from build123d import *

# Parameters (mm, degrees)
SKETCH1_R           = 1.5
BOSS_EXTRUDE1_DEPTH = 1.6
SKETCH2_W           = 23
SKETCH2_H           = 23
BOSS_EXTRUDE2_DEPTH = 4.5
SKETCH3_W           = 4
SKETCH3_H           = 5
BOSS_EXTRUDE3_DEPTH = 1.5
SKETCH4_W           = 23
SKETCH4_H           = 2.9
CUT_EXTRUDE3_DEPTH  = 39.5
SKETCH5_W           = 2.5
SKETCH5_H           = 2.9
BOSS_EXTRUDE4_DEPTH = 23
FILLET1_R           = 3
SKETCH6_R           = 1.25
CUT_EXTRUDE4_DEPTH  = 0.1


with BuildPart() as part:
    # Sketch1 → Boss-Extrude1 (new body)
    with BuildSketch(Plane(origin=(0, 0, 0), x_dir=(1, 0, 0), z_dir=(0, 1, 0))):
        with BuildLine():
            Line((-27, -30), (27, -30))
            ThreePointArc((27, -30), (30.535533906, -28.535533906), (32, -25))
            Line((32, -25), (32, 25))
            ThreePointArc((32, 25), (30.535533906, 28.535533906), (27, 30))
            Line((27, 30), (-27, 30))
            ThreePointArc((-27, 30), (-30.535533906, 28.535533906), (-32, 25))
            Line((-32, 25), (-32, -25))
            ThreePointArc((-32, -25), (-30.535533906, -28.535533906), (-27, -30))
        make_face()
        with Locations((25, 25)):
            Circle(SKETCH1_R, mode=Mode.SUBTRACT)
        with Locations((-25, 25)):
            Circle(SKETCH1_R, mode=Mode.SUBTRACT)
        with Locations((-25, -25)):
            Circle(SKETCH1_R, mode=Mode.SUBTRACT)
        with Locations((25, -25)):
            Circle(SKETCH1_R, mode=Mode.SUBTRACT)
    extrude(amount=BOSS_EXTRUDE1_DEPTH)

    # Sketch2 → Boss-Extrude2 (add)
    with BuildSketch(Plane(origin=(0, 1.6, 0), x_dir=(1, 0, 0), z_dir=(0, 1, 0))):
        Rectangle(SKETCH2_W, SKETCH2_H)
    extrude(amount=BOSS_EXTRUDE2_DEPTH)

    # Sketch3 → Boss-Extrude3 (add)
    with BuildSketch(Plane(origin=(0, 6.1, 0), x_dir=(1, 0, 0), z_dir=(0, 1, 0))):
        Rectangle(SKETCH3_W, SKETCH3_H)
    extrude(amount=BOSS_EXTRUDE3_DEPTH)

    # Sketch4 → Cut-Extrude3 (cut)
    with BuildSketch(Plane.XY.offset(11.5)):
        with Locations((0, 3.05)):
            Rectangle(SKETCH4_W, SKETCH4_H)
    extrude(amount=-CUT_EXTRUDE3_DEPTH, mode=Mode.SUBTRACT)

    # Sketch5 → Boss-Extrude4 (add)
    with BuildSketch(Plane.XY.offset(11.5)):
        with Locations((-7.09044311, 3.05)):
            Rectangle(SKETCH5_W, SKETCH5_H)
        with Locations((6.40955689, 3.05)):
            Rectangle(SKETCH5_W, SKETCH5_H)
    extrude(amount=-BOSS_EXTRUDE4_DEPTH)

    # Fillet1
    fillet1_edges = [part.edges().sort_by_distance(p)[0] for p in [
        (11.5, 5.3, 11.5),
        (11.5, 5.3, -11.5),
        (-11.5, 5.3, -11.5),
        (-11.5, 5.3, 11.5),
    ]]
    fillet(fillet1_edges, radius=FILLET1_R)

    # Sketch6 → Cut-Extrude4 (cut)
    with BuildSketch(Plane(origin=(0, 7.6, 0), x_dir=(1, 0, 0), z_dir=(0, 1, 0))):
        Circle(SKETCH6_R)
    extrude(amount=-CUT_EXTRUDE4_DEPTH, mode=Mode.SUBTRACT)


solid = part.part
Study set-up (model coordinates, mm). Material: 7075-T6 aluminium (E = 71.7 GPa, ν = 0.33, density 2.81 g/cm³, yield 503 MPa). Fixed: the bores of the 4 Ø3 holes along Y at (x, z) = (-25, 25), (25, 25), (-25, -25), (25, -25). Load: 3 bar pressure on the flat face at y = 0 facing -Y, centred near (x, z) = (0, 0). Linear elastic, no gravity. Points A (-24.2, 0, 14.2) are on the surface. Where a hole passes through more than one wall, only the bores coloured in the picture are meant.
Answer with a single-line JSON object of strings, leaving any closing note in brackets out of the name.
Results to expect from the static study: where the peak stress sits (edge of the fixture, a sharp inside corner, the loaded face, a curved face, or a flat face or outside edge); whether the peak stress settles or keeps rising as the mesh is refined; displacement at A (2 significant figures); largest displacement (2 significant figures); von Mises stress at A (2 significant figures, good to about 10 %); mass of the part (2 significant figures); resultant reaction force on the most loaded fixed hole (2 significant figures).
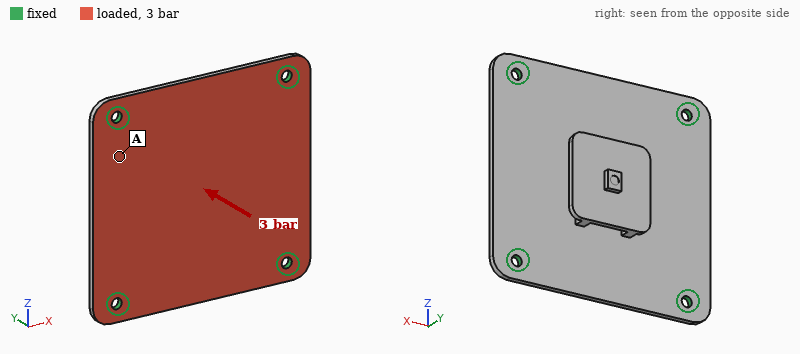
{"where the peak stress sits": "edge of the fixture", "whether the peak stress settles or keeps rising as the mesh is refined": "keeps rising", "displacement at A": "0.12 mm", "largest displacement": "0.31 mm", "von Mises stress at A": "45 MPa", "mass of the part": "20 g", "resultant reaction force on the most loaded fixed hole": "290 N"}
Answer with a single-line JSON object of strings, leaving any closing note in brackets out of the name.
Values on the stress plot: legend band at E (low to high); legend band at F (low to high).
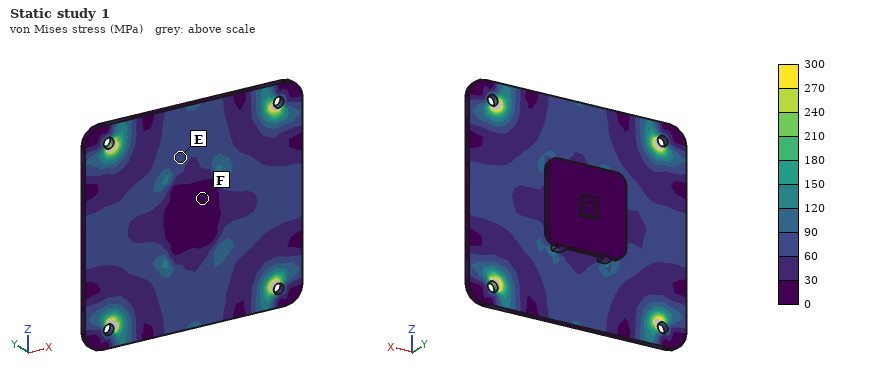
{"legend band at E": "60 to 90 MPa", "legend band at F": "0 to 30 MPa"}
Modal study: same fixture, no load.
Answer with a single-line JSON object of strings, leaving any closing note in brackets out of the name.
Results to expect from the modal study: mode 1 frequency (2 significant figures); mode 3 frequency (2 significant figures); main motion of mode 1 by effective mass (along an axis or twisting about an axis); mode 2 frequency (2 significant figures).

{"mode 1 frequency": "2200 Hz", "mode 3 frequency": "3700 Hz", "main motion of mode 1 by effective mass": "along Y", "mode 2 frequency": "3700 Hz"}
